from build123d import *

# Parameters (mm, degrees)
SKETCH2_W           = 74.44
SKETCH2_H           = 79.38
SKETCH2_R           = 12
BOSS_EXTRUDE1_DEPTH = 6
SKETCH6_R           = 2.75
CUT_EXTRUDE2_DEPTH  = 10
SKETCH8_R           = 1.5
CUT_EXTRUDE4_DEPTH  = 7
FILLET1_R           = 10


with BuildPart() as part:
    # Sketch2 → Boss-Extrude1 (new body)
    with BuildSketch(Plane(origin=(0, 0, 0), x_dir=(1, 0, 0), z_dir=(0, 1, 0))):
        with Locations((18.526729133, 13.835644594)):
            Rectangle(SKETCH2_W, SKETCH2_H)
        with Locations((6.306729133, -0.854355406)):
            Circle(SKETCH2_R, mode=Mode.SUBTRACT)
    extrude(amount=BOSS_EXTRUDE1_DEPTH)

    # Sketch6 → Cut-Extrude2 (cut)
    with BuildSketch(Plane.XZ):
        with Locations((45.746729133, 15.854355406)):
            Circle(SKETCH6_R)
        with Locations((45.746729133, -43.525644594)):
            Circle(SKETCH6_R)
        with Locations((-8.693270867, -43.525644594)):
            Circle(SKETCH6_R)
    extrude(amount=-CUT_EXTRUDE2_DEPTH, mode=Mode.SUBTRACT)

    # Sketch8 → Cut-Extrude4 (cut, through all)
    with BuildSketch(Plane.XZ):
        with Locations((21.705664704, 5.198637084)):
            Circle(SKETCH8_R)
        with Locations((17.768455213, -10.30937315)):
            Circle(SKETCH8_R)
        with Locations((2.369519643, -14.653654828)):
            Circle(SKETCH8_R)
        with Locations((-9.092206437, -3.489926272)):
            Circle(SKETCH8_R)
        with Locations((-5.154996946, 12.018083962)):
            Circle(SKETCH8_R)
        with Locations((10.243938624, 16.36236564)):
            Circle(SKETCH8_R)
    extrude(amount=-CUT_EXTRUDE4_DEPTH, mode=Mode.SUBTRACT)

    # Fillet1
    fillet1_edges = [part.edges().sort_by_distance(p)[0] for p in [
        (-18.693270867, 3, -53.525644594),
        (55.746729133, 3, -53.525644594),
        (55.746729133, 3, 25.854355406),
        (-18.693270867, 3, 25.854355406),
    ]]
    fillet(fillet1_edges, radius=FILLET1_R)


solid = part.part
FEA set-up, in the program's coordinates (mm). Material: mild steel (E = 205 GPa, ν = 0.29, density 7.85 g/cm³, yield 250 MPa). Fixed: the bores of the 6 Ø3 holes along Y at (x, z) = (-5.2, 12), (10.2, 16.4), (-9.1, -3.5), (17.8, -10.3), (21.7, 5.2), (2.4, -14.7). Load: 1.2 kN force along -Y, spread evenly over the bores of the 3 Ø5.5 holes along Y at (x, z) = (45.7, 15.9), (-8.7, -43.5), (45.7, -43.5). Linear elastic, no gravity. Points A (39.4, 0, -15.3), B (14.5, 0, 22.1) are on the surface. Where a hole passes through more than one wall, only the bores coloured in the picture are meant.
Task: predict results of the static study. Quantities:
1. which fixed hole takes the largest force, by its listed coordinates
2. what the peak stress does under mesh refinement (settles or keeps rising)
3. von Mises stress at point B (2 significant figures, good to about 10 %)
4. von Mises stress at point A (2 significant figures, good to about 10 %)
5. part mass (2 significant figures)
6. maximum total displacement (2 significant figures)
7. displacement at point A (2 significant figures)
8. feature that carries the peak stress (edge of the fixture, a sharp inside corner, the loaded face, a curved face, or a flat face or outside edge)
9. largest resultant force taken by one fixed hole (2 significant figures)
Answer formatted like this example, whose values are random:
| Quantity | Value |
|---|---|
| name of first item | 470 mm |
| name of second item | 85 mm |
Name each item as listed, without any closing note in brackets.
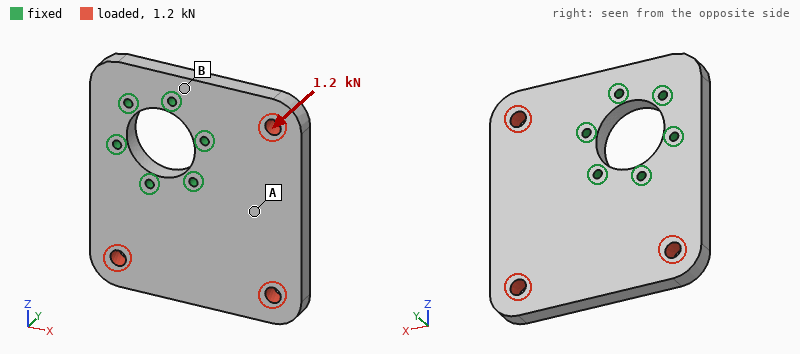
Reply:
| Quantity | Value |
|---|---|
| which fixed hole takes the largest force, by its listed coordinates | (17.8, -10.3) |
| what the peak stress does under mesh refinement | keeps rising |
| von Mises stress at point B | 14 MPa |
| von Mises stress at point A | 31 MPa |
| part mass | 250 g |
| maximum total displacement | 91 µm |
| displacement at point A | 22 µm |
| feature that carries the peak stress | edge of the fixture |
| largest resultant force taken by one fixed hole | 650 N |
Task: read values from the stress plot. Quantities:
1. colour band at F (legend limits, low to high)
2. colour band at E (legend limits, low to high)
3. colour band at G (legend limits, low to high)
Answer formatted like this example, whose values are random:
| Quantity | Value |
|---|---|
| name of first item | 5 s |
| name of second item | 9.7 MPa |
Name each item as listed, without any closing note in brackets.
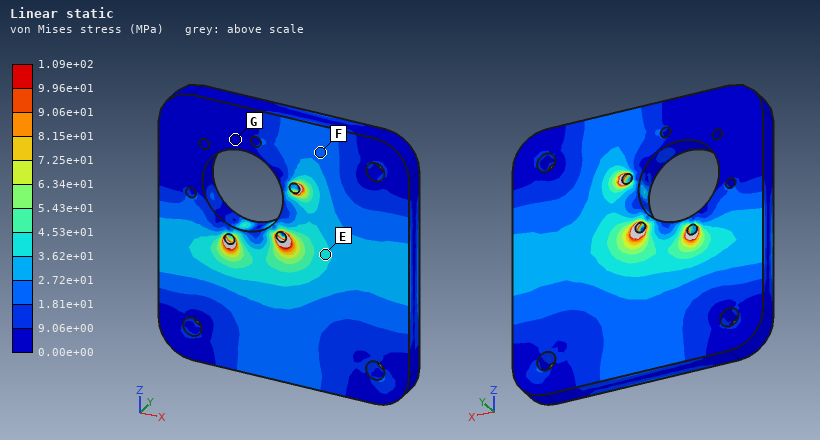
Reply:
| Quantity | Value |
|---|---|
| colour band at F | 1.81e+01 to 2.72e+01 MPa |
| colour band at E | 3.62e+01 to 4.53e+01 MPa |
| colour band at G | 0.00e+00 to 9.06e+00 MPa |
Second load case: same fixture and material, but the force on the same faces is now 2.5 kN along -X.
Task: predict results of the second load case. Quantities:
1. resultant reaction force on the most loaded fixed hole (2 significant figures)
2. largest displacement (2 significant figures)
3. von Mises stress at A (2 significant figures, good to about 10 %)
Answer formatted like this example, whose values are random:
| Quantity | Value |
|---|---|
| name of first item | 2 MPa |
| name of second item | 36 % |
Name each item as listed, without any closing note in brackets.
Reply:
| Quantity | Value |
|---|---|
| resultant reaction force on the most loaded fixed hole | 1.2 kN |
| largest displacement | 5.4 µm |
| von Mises stress at A | 4.3 MPa |
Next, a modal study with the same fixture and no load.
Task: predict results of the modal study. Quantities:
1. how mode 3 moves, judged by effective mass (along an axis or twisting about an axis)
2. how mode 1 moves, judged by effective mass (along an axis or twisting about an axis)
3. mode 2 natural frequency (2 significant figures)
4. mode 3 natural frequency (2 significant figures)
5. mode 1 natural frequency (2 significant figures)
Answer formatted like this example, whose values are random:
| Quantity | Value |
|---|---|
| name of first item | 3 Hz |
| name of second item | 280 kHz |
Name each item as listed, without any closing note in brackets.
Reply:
| Quantity | Value |
|---|---|
| how mode 3 moves, judged by effective mass | along Y |
| how mode 1 moves, judged by effective mass | along Y |
| mode 2 natural frequency | 3300 Hz |
| mode 3 natural frequency | 4600 Hz |
| mode 1 natural frequency | 2200 Hz |
